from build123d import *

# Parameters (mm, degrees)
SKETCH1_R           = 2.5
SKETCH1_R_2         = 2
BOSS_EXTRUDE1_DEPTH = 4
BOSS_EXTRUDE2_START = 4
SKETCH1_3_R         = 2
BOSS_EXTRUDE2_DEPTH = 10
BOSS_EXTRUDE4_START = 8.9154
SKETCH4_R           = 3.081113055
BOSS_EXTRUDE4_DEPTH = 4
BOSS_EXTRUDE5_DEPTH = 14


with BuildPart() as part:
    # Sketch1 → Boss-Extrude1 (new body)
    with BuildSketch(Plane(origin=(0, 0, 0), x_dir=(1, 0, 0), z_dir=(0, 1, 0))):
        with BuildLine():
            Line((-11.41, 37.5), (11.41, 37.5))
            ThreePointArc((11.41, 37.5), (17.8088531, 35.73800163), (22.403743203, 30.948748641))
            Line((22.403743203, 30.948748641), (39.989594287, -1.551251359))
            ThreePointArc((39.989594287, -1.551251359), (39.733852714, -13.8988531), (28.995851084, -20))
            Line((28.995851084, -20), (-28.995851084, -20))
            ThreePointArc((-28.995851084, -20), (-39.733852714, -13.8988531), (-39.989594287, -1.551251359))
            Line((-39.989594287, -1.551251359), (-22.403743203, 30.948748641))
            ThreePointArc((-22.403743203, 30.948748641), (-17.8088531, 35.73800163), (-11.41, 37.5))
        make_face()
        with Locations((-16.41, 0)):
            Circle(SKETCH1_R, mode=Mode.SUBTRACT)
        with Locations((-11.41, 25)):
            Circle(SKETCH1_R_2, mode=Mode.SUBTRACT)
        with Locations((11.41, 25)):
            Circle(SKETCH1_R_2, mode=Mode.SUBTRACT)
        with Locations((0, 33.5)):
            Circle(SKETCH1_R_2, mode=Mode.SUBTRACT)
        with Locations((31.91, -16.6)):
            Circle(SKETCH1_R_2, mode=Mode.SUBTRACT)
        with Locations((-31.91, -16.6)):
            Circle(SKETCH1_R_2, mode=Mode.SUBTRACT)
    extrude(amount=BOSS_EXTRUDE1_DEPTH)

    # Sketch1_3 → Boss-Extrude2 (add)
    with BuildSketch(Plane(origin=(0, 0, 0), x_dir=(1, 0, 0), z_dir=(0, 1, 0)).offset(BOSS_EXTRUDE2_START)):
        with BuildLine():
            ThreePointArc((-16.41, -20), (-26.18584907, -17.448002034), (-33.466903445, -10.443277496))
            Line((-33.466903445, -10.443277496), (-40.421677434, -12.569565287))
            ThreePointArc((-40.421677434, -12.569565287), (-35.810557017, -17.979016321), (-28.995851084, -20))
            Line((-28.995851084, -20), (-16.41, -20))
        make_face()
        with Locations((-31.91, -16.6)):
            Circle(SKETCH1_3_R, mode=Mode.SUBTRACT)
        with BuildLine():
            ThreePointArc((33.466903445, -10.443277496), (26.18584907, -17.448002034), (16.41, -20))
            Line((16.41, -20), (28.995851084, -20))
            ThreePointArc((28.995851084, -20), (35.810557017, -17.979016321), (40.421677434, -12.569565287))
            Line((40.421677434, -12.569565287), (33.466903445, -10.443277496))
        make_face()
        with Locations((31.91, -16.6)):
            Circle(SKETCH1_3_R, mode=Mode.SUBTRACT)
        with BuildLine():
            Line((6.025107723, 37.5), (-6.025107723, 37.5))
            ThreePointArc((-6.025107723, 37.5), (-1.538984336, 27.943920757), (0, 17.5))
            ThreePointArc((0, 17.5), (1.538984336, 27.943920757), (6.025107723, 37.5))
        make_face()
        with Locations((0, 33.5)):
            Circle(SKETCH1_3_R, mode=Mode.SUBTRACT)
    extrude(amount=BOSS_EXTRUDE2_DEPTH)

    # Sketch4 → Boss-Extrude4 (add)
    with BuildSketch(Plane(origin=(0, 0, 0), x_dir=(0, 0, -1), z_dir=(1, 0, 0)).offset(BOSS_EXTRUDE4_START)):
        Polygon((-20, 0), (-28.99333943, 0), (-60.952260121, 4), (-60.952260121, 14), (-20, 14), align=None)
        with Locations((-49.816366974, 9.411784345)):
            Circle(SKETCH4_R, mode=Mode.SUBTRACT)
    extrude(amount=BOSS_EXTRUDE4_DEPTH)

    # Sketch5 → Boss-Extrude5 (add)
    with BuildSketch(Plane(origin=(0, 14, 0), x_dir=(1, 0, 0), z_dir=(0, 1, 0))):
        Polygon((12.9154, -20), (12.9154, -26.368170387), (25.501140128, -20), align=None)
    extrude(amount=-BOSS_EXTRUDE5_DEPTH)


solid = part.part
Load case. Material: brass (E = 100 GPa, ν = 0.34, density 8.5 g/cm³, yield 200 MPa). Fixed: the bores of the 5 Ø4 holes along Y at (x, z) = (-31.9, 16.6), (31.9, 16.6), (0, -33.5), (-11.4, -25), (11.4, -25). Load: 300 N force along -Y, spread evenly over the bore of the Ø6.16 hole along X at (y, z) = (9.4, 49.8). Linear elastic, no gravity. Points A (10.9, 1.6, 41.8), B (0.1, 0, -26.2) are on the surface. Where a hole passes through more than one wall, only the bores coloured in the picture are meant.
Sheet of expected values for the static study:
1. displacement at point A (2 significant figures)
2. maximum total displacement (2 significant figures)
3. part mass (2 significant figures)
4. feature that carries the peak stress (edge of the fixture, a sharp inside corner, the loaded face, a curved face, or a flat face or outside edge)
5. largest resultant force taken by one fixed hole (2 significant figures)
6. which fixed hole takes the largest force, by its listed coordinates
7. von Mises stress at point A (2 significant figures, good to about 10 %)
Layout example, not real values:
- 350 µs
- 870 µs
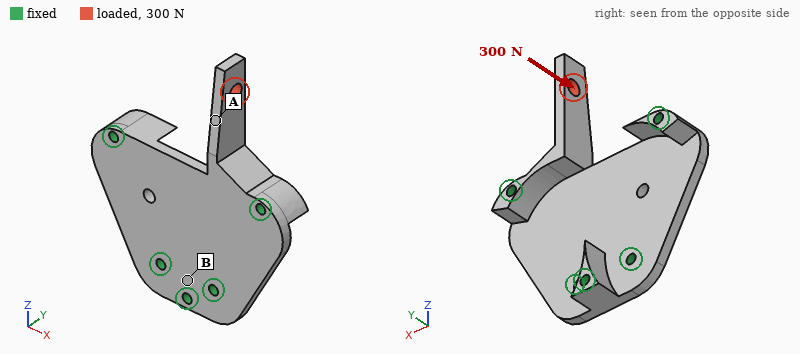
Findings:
- 0.14 mm
- 0.29 mm
- 160 g
- a curved face
- 470 N
- (31.9, 16.6)
- 27 MPa
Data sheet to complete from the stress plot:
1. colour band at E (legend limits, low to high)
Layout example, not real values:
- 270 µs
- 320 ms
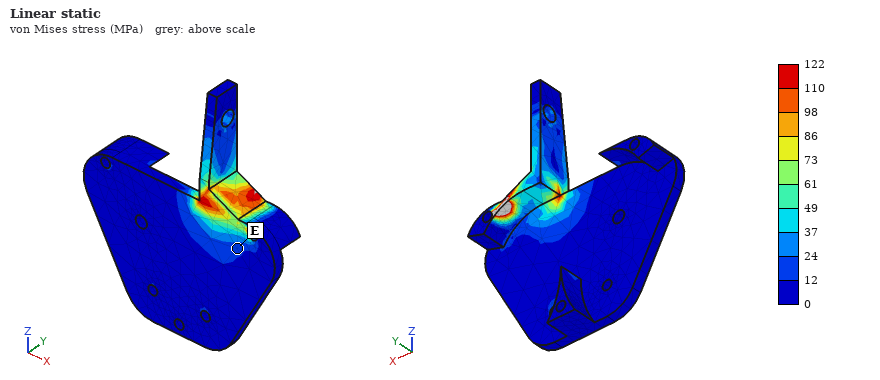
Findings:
- 12 to 24 MPa
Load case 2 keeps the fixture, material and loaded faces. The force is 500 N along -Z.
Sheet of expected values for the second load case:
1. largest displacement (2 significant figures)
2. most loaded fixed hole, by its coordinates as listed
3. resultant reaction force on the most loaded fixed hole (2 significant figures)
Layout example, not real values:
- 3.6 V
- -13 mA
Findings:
- 0.12 mm
- (31.9, 16.6)
- 200 N
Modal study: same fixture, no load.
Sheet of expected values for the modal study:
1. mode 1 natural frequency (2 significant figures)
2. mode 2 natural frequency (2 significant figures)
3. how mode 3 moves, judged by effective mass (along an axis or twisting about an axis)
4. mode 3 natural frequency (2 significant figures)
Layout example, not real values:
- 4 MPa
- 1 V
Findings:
- 1700 Hz
- 2100 Hz
- along Y
- 5000 Hz
